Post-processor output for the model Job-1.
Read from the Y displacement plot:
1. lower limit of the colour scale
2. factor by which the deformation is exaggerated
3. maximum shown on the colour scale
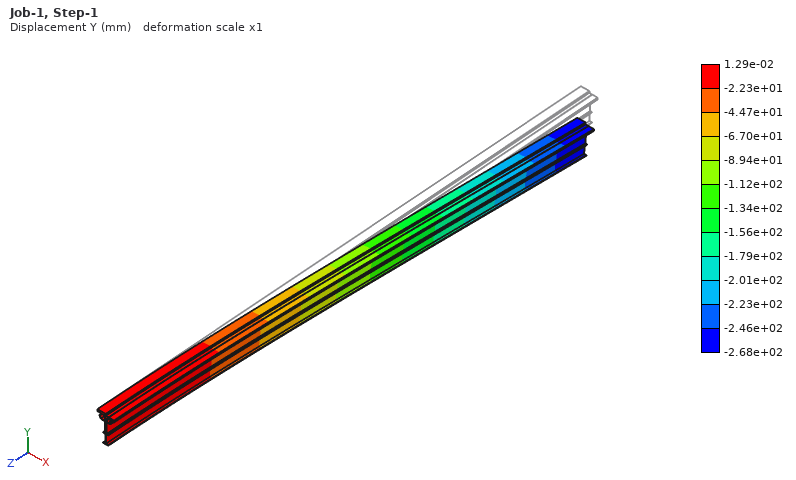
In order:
-2.68e+02 mm
1
1.29e-02 mm
